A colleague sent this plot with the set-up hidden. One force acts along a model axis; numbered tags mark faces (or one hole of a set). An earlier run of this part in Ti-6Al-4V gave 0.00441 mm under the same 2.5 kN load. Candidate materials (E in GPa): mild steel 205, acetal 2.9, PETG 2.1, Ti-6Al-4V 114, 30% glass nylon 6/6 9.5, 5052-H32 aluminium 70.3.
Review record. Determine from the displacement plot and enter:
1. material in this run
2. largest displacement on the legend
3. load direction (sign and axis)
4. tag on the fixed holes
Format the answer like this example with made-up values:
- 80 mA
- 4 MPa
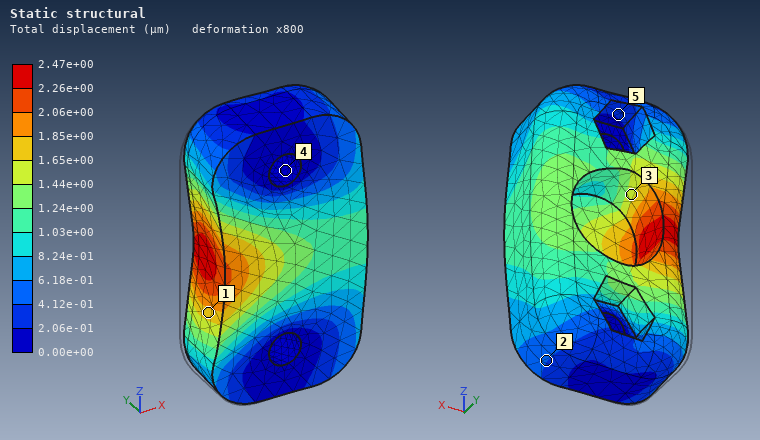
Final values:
- mild steel
- 2.47e+00 µm
- +X
- 4
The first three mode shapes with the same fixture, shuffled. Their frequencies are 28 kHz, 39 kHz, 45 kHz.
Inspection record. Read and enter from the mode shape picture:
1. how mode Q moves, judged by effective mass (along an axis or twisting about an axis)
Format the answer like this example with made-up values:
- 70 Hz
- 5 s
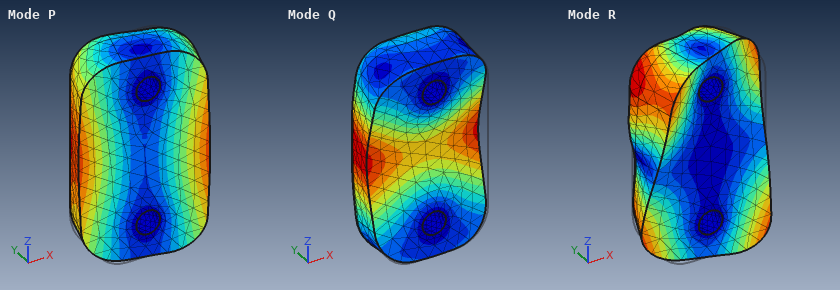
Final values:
- along Y
